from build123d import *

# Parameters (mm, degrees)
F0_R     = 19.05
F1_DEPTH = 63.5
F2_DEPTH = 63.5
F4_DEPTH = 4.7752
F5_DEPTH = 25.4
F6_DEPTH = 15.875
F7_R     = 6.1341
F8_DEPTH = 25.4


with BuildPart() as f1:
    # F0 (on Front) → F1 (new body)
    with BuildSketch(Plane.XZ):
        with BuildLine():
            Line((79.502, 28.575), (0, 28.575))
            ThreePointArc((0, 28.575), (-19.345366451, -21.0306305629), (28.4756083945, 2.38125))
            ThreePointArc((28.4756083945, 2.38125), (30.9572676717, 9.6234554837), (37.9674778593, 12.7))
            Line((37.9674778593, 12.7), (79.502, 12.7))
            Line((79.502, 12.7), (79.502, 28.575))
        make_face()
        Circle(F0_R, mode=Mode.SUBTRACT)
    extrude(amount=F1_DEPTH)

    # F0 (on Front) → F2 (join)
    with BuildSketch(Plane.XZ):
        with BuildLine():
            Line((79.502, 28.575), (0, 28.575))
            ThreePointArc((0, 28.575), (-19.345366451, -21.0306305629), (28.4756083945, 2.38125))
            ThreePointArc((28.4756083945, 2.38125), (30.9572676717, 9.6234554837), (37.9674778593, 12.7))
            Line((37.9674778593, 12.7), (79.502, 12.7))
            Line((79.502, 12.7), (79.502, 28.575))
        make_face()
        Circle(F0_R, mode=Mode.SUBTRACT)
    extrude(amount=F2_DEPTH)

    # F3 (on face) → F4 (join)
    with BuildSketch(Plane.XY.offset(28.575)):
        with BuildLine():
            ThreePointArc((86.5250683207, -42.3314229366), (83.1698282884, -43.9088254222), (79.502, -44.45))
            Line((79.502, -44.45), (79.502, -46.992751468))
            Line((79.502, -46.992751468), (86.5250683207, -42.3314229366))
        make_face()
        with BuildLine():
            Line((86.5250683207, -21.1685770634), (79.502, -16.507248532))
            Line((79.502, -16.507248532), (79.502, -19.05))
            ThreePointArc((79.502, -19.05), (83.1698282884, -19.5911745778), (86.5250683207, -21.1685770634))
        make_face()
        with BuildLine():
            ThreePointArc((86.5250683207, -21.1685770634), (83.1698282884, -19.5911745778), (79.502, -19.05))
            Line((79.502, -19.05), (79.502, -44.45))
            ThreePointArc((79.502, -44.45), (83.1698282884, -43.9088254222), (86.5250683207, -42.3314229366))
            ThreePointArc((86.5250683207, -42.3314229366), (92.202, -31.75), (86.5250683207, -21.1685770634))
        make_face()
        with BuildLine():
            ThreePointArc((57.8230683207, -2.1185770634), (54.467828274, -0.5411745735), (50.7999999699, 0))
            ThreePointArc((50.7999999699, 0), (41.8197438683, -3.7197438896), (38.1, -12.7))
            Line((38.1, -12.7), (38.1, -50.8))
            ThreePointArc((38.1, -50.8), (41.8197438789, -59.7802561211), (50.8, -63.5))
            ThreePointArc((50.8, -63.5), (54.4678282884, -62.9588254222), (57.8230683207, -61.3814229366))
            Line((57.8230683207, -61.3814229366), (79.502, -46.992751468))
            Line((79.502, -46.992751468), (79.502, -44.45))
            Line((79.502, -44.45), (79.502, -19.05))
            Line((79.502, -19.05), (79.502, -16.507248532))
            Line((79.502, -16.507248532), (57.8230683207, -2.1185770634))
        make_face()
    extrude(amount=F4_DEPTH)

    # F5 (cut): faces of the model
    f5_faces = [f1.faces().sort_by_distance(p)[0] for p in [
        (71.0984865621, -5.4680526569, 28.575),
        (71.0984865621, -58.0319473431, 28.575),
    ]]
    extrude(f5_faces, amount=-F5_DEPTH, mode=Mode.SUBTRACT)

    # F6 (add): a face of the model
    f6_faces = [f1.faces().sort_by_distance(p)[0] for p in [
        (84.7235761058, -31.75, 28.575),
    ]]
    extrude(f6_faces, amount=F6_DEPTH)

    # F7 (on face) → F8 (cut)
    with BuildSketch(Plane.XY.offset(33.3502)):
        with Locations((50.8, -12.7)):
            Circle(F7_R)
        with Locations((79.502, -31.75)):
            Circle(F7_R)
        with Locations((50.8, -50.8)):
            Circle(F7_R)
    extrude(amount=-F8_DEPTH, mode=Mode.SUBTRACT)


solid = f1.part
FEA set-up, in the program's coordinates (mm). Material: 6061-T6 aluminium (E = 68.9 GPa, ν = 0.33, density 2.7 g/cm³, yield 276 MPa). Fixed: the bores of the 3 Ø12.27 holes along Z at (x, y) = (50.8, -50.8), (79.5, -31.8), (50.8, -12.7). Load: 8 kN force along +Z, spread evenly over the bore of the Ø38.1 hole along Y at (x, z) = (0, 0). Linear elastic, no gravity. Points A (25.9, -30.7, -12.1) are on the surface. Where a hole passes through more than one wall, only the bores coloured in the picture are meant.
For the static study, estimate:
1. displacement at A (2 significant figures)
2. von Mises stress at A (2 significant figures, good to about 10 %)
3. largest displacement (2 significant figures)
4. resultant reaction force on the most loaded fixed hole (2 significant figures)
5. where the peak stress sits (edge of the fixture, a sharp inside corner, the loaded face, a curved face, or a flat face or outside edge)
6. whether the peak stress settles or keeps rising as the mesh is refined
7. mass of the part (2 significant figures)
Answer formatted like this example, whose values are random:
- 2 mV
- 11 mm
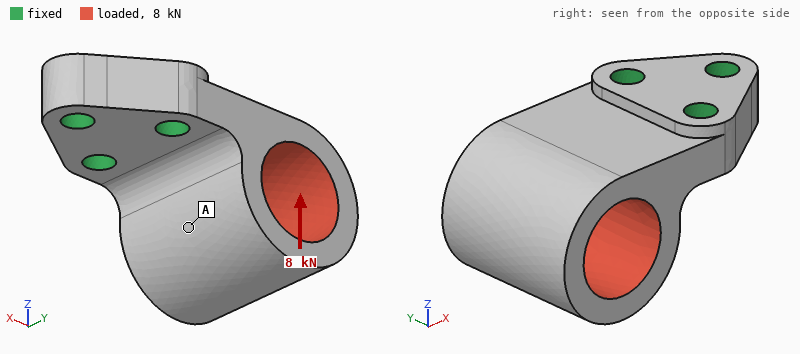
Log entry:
- 0.15 mm
- 15 MPa
- 0.34 mm
- 4.6 kN
- edge of the fixture
- keeps rising
- 420 g
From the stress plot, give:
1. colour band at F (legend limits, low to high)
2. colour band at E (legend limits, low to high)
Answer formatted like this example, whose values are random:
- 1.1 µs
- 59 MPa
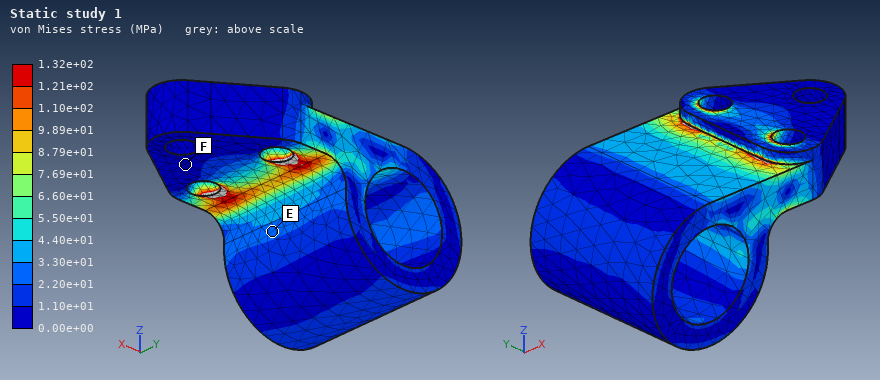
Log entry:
- 0.00e+00 to 1.10e+01 MPa
- 2.20e+01 to 3.30e+01 MPa
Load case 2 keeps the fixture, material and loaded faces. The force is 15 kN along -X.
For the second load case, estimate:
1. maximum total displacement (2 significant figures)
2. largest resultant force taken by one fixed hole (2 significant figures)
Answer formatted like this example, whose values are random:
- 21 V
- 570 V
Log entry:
- 0.39 mm
- 7.1 kN
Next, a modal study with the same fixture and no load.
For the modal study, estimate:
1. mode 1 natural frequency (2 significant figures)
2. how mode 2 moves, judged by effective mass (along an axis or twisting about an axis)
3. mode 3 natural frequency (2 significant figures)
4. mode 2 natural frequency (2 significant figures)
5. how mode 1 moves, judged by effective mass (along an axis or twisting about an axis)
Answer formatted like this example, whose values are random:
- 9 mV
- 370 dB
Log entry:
- 1600 Hz
- along Y
- 6000 Hz
- 3700 Hz
- along Z
